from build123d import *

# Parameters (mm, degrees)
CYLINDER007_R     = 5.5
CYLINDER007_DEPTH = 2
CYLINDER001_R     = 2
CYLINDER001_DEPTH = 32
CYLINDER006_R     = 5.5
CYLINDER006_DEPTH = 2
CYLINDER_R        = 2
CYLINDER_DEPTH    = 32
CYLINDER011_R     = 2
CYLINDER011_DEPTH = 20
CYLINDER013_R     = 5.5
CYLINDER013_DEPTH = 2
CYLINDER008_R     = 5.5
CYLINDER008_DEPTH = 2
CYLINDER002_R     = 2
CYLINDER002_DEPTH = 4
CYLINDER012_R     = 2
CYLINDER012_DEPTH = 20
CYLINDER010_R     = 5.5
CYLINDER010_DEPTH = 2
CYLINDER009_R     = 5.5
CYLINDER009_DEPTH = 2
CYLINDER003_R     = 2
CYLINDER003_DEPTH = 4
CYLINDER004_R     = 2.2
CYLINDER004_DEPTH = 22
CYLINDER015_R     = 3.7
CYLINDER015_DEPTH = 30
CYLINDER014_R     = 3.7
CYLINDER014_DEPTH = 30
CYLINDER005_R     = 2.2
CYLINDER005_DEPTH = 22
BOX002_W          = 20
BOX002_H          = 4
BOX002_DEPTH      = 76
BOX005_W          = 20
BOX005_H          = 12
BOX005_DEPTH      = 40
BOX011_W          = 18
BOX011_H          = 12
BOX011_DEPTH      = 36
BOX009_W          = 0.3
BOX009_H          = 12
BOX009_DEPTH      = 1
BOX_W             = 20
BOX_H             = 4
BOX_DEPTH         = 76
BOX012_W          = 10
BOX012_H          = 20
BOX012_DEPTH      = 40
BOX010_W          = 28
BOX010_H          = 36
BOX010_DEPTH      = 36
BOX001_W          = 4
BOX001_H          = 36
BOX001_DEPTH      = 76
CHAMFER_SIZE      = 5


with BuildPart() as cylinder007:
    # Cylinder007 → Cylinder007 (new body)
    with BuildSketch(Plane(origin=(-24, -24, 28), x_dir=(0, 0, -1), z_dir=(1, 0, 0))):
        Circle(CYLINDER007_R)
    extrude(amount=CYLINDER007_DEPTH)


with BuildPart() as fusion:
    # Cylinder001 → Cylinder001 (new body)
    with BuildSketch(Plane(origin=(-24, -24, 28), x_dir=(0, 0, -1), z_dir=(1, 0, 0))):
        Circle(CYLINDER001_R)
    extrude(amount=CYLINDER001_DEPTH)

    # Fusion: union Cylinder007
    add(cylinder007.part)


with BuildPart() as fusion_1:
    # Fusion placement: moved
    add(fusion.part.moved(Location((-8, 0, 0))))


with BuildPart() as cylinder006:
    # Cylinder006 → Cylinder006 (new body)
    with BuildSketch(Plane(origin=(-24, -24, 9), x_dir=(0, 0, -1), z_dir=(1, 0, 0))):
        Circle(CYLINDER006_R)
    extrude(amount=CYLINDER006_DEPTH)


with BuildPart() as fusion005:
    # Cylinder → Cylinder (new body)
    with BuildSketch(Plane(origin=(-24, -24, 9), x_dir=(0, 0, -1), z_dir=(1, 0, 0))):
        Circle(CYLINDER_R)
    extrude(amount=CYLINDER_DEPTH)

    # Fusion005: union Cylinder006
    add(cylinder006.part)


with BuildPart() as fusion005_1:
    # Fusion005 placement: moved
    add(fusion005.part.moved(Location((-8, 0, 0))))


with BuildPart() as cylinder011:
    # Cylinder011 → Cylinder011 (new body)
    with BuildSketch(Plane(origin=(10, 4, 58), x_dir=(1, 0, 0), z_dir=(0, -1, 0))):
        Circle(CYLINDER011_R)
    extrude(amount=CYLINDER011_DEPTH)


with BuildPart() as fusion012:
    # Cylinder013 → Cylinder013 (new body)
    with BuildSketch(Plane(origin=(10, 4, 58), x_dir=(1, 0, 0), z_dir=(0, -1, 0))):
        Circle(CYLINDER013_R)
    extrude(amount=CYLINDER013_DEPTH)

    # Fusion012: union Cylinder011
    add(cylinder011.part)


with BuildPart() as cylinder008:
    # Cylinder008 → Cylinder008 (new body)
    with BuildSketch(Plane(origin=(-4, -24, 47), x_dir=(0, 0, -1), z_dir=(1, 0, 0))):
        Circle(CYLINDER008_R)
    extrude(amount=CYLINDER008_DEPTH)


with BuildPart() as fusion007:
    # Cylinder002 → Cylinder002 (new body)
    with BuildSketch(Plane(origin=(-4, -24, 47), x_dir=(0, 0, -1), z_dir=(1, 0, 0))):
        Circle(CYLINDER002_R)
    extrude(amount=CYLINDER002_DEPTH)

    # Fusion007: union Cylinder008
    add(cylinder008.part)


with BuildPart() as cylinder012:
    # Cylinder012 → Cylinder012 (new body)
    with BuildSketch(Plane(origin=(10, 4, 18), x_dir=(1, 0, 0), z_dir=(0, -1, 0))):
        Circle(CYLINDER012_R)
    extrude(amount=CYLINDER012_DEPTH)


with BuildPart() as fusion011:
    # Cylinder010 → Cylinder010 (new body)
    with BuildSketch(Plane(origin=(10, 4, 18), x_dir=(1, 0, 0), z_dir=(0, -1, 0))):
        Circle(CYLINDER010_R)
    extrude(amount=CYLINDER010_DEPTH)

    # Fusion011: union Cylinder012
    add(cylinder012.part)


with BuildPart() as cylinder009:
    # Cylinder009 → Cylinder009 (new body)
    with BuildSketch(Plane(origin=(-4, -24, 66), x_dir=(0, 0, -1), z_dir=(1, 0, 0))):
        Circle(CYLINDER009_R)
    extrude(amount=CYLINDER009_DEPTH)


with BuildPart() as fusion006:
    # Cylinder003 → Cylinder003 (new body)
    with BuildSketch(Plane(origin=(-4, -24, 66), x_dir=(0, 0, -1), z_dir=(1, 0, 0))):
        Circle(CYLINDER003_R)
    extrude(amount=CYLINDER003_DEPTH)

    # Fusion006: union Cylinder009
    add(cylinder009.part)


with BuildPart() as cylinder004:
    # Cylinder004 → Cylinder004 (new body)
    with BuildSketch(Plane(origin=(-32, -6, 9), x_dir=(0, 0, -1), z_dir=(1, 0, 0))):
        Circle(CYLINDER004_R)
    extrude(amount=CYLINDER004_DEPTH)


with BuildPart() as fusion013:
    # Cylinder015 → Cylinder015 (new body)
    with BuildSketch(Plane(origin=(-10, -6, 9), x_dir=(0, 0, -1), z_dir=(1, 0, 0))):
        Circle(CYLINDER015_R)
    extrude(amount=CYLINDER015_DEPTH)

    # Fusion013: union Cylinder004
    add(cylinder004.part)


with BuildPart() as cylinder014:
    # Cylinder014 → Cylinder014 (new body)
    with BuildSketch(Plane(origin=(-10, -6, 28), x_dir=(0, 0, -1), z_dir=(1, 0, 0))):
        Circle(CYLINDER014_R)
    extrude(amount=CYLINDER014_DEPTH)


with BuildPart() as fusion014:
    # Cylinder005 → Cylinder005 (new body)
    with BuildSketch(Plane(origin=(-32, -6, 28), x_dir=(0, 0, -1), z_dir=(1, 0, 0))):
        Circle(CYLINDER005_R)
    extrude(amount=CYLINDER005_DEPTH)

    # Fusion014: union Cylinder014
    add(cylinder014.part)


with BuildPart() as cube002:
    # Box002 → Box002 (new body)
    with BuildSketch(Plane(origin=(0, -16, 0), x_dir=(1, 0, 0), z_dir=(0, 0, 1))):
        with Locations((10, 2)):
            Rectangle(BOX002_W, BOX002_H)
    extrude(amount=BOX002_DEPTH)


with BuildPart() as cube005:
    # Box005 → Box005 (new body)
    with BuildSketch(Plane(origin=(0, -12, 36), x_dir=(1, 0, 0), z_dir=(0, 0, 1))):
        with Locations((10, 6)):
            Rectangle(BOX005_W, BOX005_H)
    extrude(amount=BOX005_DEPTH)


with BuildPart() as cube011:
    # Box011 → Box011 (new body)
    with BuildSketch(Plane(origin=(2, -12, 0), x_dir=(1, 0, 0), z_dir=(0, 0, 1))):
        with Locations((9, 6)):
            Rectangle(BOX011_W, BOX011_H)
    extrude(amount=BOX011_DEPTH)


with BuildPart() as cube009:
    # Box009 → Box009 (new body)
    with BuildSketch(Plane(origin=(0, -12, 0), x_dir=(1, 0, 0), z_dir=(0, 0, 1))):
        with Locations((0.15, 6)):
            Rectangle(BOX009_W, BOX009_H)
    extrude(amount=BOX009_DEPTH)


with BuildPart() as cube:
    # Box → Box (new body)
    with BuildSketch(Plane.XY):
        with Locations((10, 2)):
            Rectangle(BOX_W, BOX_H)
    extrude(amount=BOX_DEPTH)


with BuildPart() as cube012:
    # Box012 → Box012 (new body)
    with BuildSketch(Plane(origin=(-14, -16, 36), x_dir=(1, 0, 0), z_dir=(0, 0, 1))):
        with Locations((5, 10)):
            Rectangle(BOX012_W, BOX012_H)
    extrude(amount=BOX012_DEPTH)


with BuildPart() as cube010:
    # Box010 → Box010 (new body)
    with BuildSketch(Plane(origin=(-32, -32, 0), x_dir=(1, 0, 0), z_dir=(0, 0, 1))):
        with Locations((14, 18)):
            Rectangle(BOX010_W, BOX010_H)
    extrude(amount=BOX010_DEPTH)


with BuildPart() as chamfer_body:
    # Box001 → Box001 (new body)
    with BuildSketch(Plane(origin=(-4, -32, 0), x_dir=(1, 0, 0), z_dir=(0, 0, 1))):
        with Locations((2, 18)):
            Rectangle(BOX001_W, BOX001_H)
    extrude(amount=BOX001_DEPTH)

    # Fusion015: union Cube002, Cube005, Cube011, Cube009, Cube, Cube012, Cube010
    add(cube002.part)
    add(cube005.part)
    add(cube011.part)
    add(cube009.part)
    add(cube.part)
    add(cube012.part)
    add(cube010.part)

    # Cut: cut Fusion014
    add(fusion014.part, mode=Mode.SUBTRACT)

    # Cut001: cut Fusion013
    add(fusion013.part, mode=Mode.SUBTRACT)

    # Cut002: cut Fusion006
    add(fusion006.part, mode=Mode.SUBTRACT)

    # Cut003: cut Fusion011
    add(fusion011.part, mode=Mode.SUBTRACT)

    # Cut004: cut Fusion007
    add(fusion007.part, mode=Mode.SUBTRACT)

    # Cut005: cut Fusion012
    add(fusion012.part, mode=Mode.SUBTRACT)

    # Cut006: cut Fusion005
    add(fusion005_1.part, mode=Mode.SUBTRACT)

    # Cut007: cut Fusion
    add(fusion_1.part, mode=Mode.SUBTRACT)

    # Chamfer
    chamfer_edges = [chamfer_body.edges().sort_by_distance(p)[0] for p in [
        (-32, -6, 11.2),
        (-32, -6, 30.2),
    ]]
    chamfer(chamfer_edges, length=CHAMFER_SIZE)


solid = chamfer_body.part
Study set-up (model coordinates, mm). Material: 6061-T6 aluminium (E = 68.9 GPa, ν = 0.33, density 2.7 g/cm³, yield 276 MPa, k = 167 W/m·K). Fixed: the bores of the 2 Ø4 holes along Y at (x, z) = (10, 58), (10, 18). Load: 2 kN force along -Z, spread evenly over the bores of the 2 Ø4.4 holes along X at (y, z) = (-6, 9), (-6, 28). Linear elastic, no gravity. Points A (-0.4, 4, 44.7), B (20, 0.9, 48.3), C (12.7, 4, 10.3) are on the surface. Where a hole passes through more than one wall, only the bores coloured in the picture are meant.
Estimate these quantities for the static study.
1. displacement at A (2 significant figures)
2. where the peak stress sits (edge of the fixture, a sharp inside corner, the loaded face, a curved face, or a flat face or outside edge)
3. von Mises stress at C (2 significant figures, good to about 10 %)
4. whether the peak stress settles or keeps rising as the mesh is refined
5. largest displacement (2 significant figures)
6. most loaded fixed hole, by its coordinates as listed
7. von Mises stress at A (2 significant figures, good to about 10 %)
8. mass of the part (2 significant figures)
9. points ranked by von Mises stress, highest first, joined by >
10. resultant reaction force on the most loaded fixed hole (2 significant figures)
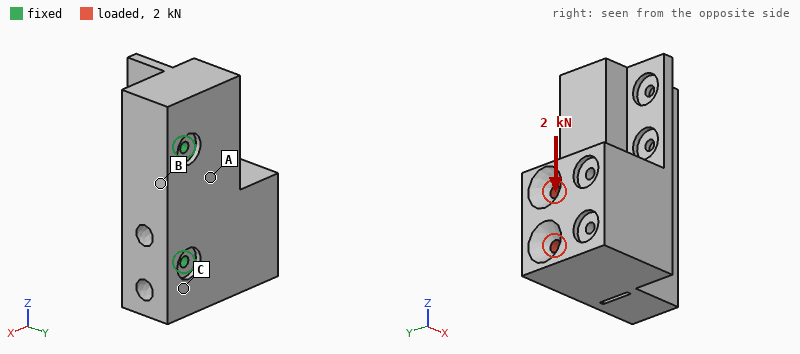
1.4 µm
edge of the fixture
3.0 MPa
keeps rising
9.6 µm
(10, 58)
5.6 MPa
210 g
A > C > B
1.8 kN
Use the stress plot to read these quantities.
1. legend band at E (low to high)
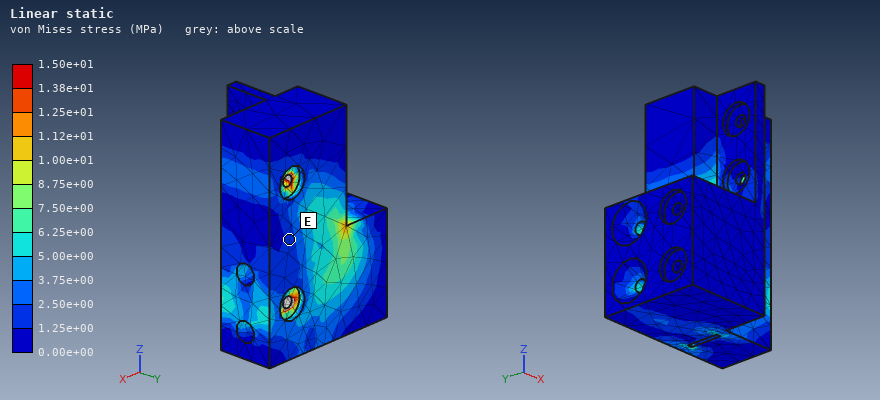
1.25e+00 to 2.50e+00 MPa
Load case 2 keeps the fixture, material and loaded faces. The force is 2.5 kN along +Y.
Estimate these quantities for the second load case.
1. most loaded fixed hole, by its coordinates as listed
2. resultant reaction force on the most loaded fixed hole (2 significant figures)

(10, 18)
2.1 kN
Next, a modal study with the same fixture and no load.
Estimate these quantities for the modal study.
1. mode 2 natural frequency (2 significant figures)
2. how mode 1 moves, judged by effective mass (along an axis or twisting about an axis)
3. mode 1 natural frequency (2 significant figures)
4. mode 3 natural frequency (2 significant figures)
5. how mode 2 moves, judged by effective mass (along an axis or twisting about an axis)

8100 Hz
along Y
4400 Hz
11 kHz
along Z
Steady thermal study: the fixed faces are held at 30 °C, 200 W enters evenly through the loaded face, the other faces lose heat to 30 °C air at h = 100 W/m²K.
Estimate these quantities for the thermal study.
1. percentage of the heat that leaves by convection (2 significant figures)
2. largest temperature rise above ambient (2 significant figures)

19 %
50 K
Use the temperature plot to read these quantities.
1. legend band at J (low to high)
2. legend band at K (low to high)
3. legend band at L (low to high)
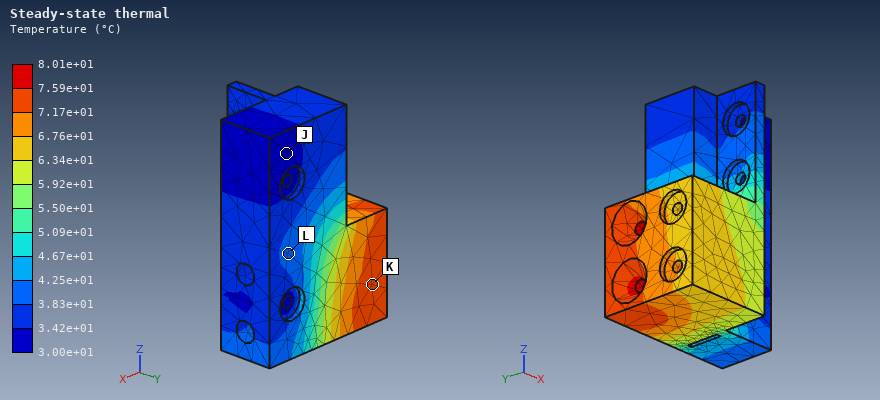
3.00e+01 to 3.42e+01 °C
7.17e+01 to 7.59e+01 °C
3.83e+01 to 4.25e+01 °C
